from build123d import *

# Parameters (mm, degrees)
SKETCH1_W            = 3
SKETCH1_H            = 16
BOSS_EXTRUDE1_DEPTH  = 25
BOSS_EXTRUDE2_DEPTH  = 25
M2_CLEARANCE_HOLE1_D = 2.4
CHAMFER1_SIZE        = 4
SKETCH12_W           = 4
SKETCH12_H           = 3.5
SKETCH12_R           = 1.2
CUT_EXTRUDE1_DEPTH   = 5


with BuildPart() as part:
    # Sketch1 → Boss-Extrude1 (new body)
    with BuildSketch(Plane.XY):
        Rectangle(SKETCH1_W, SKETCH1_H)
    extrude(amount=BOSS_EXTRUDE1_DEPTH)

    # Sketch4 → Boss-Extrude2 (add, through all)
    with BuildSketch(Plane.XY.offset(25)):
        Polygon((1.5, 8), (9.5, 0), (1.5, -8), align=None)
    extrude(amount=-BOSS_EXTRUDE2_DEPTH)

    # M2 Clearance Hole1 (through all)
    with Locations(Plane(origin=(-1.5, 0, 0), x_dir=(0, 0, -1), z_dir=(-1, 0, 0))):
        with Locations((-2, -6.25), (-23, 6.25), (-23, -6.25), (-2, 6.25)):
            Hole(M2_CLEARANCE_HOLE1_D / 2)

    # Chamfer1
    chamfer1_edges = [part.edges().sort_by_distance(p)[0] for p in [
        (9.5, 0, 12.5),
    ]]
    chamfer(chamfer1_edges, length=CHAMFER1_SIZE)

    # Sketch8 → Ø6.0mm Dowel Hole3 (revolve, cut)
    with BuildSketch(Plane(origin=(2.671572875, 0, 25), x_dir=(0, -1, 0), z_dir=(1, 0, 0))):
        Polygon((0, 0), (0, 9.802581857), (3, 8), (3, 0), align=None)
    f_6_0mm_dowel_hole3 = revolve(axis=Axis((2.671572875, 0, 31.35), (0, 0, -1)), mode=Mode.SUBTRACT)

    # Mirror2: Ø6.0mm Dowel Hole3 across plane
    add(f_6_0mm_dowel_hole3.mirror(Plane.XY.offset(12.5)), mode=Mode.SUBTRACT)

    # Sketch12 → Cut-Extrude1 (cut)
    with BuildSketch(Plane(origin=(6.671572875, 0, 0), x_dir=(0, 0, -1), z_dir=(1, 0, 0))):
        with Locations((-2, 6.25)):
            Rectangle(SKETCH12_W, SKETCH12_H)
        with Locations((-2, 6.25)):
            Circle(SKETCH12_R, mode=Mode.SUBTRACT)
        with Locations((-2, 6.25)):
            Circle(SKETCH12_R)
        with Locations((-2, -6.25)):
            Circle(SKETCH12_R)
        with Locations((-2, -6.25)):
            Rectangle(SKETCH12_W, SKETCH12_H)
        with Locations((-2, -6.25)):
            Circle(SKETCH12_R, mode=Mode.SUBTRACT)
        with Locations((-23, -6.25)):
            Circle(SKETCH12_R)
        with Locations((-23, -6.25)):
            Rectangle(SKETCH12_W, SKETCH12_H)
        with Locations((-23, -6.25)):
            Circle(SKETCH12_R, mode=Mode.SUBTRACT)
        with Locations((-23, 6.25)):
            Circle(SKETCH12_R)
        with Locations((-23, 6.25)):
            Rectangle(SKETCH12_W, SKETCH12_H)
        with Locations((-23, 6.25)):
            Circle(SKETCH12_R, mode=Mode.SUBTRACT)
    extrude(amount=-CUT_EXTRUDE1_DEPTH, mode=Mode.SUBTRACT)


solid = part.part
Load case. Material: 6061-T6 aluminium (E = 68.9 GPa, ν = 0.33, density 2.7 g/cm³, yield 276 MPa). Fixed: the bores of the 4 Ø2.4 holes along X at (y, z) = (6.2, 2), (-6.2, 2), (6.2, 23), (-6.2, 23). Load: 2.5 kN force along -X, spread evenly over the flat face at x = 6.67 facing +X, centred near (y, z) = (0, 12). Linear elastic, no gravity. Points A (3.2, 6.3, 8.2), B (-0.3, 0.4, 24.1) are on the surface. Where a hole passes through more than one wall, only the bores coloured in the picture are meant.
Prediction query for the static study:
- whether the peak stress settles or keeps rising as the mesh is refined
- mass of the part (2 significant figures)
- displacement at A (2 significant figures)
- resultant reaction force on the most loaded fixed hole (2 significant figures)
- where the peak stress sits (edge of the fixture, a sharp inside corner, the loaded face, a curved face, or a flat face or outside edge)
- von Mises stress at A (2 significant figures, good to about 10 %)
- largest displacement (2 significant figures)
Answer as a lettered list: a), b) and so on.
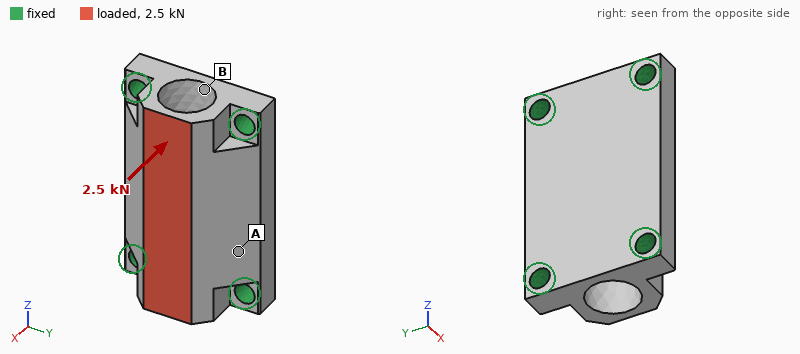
a) keeps rising
b) 5.3 g
c) 6.7 µm
d) 690 N
e) edge of the fixture
f) 23 MPa
g) 11 µm
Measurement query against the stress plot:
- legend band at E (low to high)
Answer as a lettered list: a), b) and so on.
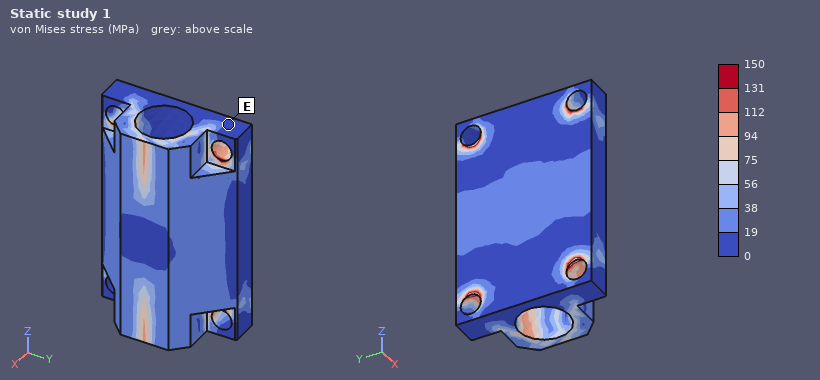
a) 0 to 19 MPa
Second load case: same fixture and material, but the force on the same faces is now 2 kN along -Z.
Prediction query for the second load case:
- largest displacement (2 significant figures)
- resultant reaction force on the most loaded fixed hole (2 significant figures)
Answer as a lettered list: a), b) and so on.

a) 12 µm
b) 610 N
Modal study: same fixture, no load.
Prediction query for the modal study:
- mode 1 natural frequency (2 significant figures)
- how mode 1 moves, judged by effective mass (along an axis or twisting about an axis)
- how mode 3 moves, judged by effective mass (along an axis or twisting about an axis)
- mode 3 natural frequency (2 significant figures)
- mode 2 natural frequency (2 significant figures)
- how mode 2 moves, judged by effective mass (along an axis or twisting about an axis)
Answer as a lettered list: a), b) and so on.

a) 38 kHz
b) along X
c) along Y
d) 53 kHz
e) 43 kHz
f) along Y
